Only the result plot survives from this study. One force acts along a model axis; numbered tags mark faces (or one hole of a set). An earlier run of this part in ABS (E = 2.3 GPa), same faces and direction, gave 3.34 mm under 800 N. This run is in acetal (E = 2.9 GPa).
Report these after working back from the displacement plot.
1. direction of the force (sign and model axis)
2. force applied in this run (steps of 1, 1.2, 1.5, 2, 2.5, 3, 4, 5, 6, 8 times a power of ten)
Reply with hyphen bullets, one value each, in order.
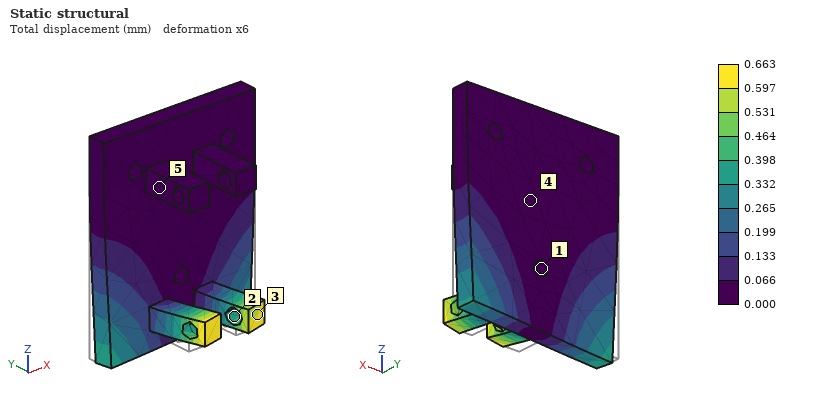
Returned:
- +X
- 200 N
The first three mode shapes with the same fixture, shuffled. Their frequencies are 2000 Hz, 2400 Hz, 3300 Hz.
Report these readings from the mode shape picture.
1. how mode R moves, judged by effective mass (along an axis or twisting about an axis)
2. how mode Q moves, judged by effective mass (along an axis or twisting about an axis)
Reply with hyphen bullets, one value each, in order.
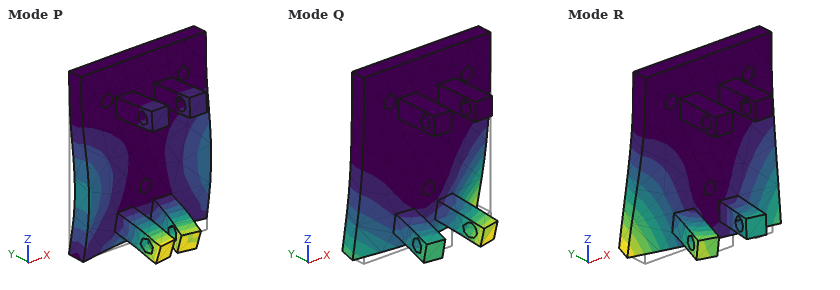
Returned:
- twisting about Z
- along Y
